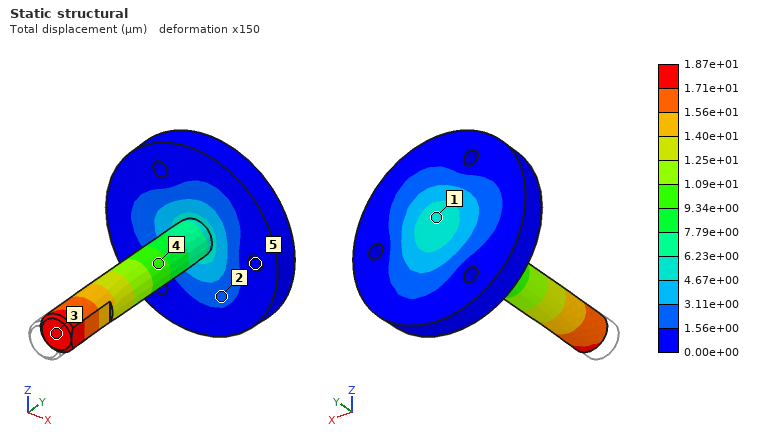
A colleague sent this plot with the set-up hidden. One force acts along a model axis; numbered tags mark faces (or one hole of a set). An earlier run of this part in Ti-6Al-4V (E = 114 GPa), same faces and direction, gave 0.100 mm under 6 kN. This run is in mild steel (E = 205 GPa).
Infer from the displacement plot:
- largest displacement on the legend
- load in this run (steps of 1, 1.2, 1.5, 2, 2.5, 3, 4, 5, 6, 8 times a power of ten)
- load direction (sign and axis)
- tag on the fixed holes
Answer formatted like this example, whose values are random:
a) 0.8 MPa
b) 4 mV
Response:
a) 1.87e+01 µm
b) 2 kN
c) +Y
d) 5
